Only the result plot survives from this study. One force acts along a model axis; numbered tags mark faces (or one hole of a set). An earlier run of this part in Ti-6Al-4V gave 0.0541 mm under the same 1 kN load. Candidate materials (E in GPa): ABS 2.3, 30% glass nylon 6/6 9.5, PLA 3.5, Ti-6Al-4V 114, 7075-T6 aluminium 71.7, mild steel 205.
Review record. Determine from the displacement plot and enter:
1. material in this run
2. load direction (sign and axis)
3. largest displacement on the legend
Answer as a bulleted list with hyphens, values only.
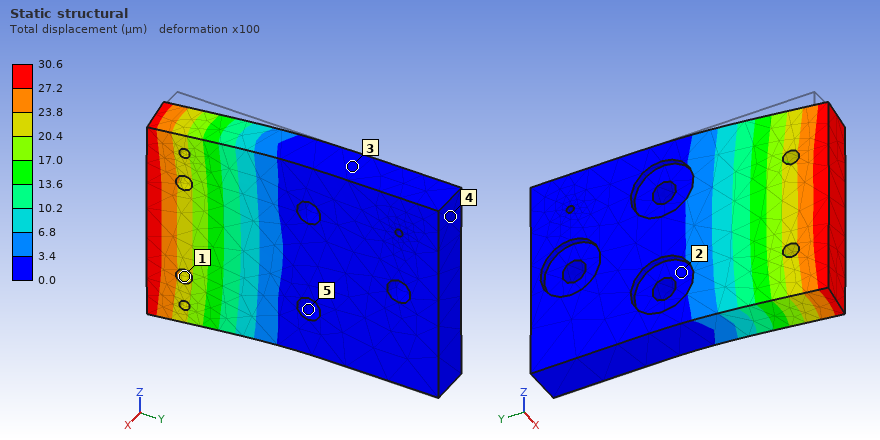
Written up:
- mild steel
- +X
- 30.6 µm
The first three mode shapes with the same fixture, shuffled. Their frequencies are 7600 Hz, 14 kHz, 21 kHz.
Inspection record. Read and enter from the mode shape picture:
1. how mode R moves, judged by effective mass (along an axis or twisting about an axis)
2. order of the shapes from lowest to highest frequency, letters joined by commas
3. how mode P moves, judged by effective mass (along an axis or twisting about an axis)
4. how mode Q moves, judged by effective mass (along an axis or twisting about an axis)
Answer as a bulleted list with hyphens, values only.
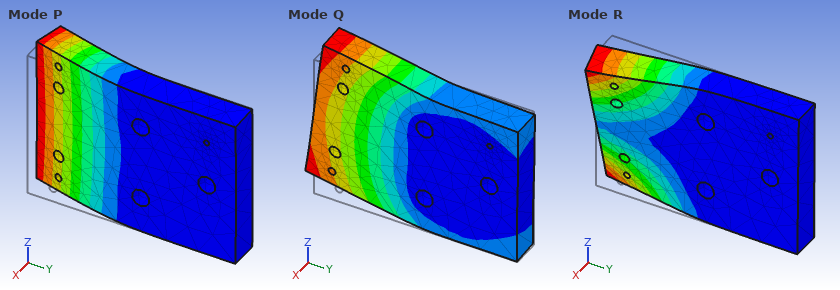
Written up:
- twisting about Y
- P, R, Q
- along X
- along Z
